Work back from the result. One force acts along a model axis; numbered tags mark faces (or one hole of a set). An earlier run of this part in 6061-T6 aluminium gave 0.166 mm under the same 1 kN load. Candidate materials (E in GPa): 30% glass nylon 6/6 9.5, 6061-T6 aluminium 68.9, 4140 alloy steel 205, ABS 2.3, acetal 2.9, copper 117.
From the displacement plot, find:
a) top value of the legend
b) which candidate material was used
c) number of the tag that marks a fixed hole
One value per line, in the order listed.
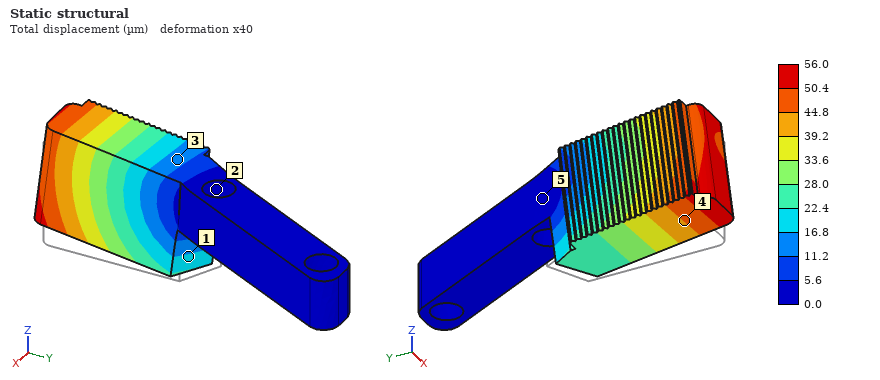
56.0 µm
4140 alloy steel
2
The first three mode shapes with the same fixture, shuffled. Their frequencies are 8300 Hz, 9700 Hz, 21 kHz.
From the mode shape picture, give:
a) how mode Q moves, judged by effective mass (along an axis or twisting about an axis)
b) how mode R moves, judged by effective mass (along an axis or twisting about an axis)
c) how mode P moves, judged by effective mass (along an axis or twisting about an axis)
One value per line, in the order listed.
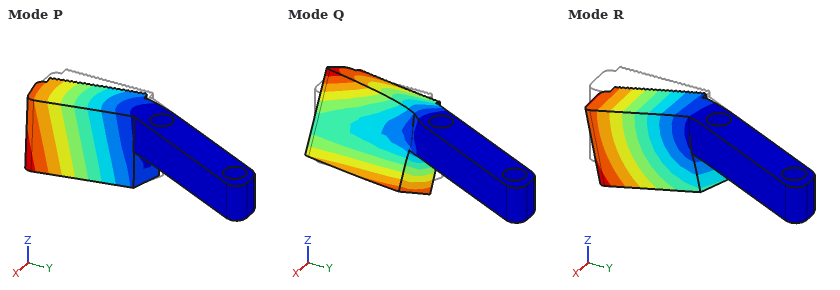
twisting about Y
along Z
along X
